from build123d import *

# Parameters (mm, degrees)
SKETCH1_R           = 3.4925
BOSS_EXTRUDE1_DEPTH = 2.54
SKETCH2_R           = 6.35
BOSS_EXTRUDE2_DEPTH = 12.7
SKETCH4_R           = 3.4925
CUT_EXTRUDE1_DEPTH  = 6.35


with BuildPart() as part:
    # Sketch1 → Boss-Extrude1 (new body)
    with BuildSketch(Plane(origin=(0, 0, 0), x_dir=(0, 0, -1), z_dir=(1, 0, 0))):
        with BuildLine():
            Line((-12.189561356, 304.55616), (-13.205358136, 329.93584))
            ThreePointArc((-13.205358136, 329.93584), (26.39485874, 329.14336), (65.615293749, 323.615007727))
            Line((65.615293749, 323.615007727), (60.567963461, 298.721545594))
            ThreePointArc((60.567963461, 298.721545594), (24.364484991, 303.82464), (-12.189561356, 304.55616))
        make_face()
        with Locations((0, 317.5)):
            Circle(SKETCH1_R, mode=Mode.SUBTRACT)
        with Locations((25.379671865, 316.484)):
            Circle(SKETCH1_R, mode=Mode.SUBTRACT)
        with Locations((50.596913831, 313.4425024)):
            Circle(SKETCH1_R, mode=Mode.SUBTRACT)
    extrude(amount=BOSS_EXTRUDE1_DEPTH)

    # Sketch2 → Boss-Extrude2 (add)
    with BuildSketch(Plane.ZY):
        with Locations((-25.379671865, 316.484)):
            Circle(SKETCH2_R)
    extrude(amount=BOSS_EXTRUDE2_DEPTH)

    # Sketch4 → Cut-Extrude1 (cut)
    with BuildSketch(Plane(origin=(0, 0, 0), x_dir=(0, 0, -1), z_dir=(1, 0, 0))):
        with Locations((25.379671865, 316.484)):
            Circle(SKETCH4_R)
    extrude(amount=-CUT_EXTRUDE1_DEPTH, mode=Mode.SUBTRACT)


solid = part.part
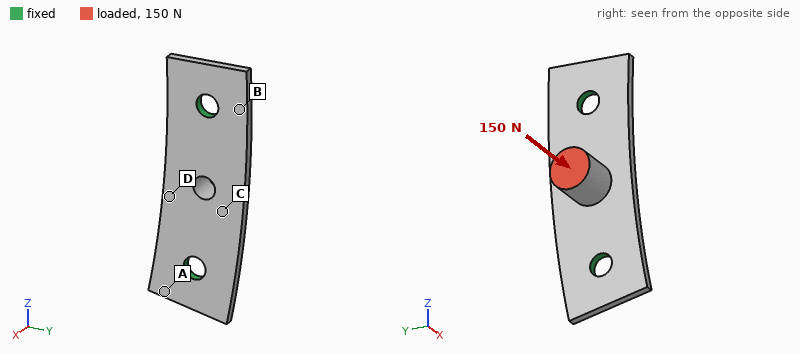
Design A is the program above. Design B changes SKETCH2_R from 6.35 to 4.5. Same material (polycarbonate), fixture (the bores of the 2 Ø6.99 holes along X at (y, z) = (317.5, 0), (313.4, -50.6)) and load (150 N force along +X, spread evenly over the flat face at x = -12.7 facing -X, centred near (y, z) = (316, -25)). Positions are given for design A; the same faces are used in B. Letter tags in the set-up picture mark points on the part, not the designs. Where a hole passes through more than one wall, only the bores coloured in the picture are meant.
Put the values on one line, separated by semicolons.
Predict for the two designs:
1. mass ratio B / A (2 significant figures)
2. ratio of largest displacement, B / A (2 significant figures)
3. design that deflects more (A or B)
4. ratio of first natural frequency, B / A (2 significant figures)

0.87; 1.3; B; 1.1
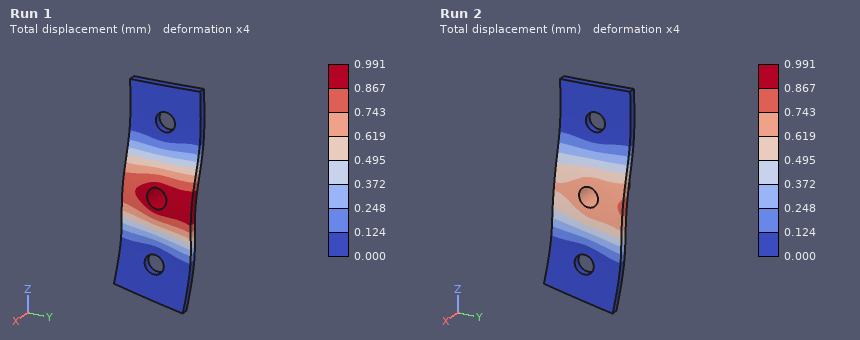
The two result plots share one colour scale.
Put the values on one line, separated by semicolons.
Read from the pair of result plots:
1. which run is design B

Run 1
